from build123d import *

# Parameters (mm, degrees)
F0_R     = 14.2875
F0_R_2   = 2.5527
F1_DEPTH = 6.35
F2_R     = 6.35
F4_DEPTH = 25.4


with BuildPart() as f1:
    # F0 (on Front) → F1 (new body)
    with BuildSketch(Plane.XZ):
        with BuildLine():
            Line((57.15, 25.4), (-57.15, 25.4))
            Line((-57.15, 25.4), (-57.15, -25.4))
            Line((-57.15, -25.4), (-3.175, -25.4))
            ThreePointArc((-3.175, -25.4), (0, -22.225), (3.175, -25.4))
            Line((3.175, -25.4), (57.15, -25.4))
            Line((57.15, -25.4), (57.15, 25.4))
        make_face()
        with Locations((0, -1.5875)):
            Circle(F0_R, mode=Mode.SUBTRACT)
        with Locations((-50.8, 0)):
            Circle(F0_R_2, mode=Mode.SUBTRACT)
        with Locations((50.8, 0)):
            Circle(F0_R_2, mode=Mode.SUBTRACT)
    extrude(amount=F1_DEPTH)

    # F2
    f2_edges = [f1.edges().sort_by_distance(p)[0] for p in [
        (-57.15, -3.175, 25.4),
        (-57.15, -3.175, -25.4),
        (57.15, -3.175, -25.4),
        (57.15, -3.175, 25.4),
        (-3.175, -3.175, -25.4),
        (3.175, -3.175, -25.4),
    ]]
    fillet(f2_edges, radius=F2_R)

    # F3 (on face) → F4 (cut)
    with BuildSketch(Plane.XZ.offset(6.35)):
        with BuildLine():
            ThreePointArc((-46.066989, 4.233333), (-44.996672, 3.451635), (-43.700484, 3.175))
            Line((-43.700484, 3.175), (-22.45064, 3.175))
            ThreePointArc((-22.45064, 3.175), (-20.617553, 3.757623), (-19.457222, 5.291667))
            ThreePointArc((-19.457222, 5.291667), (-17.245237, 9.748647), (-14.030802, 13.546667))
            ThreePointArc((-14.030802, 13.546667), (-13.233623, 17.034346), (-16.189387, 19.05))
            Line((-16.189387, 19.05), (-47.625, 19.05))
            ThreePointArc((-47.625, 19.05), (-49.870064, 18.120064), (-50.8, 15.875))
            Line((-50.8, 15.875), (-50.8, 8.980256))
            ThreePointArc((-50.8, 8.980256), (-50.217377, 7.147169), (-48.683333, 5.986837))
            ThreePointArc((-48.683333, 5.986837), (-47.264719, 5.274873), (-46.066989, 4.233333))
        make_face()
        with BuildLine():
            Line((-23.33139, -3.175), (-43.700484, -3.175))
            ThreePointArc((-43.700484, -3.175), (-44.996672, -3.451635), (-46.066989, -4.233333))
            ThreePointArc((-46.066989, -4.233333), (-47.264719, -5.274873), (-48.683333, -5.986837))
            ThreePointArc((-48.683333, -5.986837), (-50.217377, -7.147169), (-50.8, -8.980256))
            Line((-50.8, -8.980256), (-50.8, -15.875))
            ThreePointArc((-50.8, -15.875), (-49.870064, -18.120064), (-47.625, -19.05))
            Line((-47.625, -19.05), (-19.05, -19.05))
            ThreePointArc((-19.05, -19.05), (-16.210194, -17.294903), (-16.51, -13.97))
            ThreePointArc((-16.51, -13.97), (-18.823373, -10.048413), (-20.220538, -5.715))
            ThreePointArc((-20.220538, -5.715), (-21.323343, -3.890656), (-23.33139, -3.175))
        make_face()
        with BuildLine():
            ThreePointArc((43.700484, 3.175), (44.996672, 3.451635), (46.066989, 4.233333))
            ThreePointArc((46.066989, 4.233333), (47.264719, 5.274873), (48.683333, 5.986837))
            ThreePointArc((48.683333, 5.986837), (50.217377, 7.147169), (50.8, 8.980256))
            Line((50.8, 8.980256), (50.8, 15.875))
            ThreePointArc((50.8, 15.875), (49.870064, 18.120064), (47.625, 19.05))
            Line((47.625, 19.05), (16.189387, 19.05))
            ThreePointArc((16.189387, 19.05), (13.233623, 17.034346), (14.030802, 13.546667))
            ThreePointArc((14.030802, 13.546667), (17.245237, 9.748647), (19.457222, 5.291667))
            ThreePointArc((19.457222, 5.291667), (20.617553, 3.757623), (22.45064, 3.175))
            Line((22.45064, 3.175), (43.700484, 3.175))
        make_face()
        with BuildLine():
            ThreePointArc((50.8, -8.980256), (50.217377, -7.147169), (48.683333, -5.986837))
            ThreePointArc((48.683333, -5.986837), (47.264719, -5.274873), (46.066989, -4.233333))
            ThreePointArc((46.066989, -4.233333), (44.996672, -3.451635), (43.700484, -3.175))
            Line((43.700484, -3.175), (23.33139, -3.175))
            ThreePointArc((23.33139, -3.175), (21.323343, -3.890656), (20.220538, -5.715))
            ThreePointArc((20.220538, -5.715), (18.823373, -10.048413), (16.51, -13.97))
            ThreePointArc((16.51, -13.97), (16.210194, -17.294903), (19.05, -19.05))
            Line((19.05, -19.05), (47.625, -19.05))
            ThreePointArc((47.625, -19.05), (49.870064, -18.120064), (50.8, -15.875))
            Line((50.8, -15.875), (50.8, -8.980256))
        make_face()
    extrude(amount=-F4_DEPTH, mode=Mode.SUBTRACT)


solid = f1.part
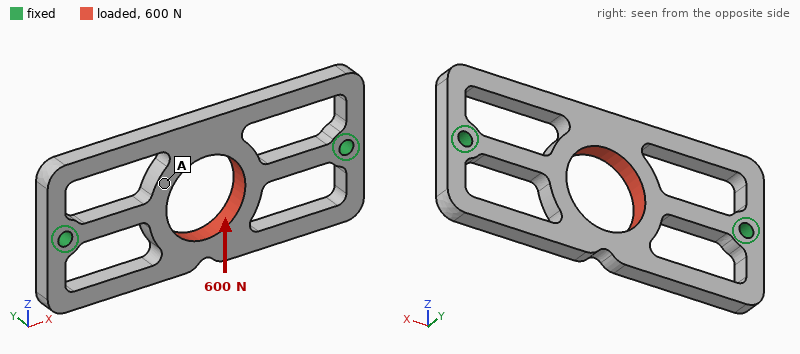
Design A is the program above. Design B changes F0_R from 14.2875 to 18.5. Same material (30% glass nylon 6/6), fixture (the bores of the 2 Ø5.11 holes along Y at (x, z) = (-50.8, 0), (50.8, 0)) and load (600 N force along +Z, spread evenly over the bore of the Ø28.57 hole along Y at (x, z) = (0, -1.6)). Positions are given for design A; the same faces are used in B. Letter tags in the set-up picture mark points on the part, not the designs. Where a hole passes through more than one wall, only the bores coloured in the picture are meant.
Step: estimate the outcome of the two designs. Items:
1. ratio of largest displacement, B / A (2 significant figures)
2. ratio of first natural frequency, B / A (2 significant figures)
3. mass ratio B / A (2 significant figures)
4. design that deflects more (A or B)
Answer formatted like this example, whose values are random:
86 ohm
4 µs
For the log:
1.8
0.99
0.86
B
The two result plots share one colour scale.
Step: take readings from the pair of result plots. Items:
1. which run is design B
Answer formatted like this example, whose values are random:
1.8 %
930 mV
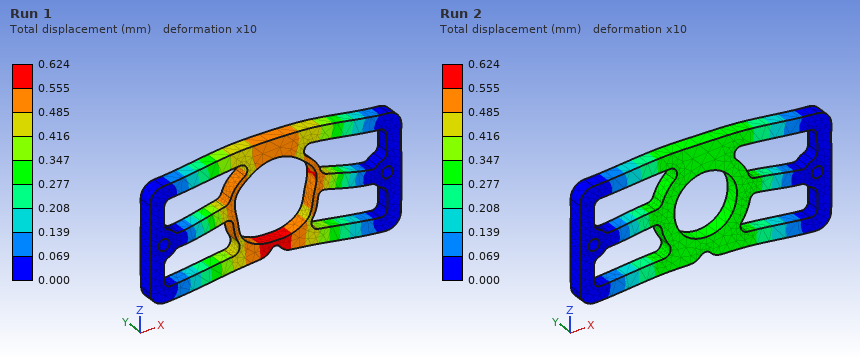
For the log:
Run 1
